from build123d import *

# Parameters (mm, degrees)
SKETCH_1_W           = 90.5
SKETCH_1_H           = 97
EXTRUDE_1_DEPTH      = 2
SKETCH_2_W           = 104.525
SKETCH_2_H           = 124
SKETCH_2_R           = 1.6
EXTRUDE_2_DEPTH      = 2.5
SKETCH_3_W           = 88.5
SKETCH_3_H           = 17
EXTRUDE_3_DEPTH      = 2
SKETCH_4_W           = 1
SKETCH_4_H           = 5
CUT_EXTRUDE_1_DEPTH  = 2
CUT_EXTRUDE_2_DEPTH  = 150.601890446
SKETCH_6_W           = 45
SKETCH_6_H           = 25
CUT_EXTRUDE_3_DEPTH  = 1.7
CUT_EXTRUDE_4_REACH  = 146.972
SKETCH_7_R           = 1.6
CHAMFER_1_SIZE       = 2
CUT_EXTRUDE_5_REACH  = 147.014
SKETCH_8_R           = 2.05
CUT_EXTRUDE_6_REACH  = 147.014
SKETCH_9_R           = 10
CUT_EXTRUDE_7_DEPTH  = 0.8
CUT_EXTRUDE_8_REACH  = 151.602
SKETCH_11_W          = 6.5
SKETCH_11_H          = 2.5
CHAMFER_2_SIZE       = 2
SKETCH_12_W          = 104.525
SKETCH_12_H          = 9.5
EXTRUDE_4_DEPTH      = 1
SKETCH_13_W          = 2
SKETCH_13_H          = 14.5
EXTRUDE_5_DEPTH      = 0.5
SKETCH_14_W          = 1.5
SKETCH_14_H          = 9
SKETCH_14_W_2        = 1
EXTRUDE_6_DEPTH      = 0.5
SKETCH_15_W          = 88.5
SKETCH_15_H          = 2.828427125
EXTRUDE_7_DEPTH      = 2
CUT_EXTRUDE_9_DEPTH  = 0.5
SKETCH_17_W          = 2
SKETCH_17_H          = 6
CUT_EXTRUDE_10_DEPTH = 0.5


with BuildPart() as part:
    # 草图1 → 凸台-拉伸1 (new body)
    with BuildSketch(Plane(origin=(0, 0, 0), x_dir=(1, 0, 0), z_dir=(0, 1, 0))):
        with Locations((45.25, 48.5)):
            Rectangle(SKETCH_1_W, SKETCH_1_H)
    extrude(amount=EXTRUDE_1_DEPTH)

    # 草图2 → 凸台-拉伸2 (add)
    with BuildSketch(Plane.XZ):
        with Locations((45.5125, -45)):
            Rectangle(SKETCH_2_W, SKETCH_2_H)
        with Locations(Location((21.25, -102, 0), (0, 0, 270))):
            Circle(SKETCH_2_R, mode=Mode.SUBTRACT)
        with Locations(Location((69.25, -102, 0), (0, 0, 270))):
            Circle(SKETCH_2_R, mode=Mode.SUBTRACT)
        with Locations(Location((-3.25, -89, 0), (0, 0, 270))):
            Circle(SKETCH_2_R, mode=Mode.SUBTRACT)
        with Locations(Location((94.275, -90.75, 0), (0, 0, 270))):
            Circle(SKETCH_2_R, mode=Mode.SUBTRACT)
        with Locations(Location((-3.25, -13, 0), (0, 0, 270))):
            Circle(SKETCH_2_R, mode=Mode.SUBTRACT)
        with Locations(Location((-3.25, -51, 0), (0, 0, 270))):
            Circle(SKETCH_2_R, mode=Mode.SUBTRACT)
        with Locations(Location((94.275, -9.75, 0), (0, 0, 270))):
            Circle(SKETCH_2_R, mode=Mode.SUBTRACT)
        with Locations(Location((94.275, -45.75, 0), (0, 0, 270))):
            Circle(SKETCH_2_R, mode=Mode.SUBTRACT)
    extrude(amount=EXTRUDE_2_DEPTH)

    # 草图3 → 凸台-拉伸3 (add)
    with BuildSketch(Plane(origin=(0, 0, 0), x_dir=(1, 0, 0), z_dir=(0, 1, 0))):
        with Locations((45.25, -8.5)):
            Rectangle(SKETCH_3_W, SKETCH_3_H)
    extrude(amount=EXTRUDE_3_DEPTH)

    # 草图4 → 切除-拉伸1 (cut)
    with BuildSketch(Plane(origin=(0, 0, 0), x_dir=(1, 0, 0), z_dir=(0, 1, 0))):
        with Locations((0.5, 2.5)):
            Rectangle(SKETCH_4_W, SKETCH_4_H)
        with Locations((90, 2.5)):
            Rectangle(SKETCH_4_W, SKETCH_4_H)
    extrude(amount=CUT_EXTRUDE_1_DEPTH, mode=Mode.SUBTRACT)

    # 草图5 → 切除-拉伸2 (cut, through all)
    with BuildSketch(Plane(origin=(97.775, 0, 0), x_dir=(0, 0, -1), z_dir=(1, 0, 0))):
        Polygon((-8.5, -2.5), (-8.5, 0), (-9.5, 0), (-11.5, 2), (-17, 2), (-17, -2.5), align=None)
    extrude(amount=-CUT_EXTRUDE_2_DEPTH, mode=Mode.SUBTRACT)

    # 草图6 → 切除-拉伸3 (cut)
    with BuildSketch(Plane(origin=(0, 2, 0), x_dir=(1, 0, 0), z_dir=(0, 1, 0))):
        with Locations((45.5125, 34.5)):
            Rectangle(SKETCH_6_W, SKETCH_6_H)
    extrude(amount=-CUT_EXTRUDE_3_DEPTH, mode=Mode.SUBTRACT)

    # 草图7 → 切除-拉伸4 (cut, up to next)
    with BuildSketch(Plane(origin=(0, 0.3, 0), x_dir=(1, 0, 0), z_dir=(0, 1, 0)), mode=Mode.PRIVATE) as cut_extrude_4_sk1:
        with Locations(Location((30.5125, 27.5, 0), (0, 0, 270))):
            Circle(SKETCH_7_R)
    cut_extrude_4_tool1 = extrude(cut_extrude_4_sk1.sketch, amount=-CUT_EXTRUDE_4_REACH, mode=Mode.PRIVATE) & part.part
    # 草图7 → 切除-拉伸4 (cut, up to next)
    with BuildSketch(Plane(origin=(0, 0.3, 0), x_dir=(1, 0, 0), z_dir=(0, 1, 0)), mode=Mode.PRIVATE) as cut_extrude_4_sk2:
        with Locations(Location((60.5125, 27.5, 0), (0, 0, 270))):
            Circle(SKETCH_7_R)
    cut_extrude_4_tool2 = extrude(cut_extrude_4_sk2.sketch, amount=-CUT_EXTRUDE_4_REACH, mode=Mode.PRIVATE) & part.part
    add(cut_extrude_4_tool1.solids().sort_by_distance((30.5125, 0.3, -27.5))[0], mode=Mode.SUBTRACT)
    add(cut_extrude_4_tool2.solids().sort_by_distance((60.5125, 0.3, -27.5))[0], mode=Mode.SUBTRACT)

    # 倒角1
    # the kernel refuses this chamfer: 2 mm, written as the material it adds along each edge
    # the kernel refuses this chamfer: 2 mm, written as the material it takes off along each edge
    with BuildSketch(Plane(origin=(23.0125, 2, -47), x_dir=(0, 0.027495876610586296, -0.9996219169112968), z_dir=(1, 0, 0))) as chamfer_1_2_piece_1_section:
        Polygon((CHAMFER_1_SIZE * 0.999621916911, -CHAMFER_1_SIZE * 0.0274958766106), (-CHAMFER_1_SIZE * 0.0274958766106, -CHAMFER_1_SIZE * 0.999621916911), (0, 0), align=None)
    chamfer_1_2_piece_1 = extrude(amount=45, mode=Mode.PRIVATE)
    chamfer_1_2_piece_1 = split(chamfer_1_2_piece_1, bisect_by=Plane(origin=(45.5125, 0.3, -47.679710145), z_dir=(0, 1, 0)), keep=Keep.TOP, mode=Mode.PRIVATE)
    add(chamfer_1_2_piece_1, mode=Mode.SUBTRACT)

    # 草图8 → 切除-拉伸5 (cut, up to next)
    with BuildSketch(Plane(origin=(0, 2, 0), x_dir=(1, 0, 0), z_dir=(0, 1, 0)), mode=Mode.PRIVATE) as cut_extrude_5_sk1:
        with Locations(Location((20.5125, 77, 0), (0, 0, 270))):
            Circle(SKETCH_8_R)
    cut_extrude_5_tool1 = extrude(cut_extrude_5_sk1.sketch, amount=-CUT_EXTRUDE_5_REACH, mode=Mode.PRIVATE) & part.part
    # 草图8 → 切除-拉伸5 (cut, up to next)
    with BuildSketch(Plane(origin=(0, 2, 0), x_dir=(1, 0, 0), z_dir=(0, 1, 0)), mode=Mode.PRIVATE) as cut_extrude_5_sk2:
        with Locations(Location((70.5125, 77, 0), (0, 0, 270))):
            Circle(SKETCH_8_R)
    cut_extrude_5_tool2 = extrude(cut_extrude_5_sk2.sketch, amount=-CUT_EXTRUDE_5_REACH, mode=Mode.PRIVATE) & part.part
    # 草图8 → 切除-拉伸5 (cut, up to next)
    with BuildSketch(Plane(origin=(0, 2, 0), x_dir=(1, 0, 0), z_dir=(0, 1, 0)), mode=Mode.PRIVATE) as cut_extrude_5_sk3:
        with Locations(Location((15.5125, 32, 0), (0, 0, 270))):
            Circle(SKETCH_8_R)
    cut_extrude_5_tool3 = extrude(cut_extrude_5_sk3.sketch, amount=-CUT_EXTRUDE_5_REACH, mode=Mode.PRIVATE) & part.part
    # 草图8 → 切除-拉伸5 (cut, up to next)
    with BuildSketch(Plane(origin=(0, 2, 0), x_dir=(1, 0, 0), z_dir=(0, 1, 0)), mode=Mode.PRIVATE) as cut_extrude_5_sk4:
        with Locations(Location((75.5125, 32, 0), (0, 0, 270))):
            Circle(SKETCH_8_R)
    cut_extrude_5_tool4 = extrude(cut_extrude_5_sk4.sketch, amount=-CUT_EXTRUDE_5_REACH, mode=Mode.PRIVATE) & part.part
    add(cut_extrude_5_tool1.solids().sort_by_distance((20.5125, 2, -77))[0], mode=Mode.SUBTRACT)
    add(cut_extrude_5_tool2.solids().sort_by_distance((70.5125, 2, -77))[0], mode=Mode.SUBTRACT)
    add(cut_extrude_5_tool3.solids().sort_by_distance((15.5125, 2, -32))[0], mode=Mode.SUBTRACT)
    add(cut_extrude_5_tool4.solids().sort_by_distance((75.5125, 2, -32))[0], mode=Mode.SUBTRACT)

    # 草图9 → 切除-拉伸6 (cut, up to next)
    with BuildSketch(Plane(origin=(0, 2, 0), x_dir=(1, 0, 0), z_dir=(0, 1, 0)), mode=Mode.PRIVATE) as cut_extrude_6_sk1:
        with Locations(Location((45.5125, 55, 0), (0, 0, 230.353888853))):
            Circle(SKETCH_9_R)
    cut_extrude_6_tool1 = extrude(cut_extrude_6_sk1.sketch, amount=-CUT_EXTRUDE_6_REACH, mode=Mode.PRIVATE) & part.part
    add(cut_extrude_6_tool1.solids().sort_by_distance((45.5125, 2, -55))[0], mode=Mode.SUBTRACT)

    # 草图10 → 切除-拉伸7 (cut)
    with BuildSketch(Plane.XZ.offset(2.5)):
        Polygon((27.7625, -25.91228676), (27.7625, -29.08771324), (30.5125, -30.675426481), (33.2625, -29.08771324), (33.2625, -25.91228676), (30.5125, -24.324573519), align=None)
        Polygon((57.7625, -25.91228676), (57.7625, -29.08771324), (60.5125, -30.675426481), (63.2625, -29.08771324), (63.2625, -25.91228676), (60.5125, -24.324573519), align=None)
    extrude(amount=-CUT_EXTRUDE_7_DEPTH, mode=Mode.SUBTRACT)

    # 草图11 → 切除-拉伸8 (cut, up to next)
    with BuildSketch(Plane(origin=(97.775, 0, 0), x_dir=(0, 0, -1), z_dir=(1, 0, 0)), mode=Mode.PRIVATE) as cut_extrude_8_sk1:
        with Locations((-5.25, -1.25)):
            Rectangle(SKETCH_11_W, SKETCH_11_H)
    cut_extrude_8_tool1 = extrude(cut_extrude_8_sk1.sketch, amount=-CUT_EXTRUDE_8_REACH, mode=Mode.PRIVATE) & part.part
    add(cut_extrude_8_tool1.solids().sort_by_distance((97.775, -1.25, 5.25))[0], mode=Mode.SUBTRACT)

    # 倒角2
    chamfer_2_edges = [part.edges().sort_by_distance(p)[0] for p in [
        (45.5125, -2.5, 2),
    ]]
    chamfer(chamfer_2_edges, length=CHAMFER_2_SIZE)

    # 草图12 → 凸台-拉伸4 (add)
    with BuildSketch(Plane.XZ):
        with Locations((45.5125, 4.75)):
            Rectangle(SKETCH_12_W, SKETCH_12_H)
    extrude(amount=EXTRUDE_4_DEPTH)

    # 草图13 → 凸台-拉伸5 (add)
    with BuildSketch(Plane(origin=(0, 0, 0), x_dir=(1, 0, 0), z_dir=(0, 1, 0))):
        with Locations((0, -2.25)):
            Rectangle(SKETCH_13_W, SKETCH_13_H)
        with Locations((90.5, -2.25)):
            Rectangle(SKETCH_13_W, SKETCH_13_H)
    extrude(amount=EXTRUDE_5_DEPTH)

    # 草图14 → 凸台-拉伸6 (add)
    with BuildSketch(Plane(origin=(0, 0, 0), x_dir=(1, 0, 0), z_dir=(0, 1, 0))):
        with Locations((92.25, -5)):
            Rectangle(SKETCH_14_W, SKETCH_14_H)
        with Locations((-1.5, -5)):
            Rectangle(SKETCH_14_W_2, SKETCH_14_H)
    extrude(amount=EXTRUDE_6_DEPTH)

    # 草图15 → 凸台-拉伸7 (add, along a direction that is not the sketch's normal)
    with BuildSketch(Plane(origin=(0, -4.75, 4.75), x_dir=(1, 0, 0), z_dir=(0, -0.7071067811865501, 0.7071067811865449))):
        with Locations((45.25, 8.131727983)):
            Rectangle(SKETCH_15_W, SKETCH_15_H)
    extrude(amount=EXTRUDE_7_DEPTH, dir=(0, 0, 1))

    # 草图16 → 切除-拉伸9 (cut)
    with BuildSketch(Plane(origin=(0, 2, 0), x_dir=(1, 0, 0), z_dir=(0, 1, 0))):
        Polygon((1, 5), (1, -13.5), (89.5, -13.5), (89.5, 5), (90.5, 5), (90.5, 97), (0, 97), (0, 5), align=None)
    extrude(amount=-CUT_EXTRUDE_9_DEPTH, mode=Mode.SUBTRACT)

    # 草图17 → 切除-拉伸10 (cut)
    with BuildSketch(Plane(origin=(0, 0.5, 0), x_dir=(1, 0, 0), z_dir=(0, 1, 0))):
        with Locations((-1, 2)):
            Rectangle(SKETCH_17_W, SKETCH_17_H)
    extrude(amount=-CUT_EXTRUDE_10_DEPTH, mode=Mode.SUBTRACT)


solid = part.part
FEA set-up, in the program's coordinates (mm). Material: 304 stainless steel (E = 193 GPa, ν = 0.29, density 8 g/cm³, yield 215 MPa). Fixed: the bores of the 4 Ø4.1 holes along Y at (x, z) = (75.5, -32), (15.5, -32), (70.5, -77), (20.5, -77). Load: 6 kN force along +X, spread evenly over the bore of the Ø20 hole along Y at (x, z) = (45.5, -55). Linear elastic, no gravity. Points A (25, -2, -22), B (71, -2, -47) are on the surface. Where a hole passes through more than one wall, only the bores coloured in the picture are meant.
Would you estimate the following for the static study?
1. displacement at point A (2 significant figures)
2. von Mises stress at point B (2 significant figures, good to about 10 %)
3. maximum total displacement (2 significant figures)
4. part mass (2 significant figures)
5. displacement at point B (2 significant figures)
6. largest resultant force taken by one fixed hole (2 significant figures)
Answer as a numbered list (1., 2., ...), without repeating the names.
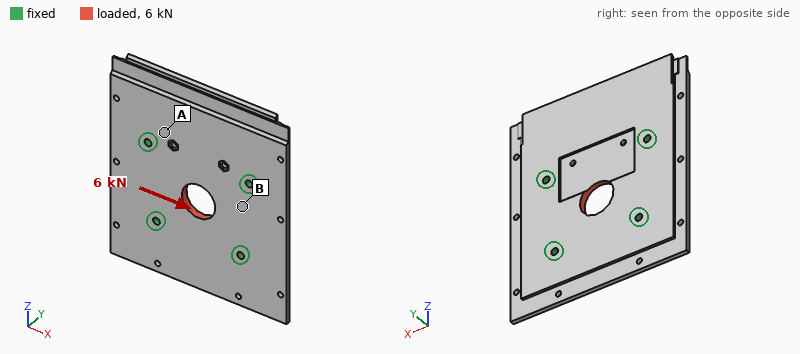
1. 0.71 µm
2. 13 MPa
3. 4.1 µm
4. 330 g
5. 2.3 µm
6. 1.7 kN
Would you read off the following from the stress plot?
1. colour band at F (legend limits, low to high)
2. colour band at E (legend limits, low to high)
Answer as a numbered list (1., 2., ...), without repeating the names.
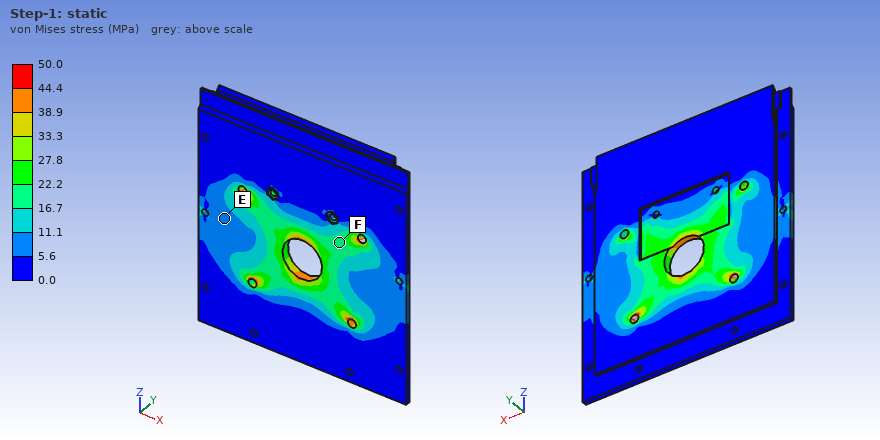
1. 16.7 to 22.2 MPa
2. 5.6 to 11.1 MPa
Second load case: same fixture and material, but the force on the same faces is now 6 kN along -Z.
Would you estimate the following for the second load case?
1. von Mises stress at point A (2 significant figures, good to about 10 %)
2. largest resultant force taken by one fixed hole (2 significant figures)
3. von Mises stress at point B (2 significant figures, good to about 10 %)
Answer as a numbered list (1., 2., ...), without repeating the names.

1. 11 MPa
2. 1.8 kN
3. 8.7 MPa
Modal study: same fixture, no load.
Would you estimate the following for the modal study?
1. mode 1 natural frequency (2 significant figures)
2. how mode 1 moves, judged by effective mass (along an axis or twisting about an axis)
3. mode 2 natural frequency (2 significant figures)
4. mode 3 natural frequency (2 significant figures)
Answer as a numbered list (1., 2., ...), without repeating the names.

1. 1500 Hz
2. along Y
3. 2400 Hz
4. 3200 Hz
